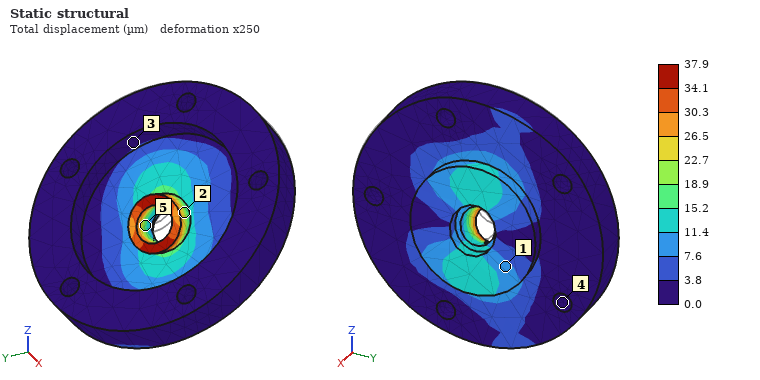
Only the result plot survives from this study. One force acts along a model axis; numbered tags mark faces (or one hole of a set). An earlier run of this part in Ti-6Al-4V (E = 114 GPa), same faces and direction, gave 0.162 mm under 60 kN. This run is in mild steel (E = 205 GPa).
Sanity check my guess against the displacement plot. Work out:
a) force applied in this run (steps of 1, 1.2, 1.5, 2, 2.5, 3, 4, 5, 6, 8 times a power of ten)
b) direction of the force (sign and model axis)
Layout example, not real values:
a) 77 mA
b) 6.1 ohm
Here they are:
a) 25 kN
b) -Z
